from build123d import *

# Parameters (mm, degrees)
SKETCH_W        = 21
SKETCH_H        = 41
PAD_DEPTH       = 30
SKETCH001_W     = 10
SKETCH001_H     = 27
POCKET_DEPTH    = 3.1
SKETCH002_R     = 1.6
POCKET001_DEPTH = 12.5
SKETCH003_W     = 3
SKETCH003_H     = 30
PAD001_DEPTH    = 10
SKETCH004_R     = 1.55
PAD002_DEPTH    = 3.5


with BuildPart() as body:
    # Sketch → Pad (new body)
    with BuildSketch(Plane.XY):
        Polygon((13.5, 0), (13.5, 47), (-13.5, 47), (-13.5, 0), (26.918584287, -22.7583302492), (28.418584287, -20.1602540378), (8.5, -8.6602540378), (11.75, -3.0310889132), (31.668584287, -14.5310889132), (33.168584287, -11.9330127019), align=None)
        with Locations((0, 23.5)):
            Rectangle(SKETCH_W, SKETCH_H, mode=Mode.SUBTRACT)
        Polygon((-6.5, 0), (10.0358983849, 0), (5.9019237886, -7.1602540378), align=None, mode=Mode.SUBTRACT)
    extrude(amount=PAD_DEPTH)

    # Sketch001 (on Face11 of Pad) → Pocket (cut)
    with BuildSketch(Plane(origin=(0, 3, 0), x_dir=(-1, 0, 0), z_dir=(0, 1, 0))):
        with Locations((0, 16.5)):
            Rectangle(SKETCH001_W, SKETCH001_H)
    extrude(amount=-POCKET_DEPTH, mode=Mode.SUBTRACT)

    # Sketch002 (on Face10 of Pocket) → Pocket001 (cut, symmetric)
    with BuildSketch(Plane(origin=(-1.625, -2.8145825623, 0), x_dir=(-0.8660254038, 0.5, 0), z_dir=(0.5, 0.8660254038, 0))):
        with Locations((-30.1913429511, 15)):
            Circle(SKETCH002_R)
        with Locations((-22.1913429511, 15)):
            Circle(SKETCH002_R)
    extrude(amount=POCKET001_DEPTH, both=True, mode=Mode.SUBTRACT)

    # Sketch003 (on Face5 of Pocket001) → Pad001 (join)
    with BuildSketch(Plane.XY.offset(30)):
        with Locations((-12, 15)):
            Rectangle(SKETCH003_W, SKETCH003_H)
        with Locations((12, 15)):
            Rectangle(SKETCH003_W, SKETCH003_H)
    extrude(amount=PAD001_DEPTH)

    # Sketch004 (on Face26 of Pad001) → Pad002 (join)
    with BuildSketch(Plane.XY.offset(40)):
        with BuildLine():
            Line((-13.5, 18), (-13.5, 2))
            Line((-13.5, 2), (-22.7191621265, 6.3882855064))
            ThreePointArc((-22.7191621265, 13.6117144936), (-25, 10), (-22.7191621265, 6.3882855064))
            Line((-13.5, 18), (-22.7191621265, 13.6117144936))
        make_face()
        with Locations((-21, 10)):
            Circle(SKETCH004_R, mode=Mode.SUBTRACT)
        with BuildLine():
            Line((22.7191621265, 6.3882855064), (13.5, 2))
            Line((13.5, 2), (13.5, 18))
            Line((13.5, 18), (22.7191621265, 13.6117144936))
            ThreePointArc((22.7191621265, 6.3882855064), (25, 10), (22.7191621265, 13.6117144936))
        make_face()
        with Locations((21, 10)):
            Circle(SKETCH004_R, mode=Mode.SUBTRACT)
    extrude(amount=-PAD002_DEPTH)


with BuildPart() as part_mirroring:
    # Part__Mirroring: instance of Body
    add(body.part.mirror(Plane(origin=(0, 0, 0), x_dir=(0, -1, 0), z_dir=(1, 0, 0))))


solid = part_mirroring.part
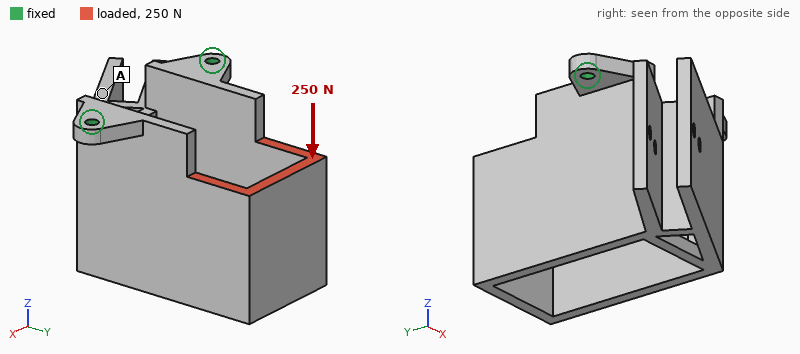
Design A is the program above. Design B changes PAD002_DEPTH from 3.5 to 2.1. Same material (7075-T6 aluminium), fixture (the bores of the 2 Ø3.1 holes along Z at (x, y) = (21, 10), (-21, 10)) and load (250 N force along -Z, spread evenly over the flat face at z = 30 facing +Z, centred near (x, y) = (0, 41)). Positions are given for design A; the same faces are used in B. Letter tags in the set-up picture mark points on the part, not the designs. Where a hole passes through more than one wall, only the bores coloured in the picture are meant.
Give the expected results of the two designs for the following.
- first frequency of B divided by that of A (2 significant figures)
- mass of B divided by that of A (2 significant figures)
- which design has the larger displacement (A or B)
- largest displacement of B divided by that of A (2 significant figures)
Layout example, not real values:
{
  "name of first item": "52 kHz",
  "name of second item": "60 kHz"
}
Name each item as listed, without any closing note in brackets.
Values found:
{
  "first frequency of B divided by that of A": "0.54",
  "mass of B divided by that of A": "0.99",
  "which design has the larger displacement": "B",
  "largest displacement of B divided by that of A": "3.3"
}
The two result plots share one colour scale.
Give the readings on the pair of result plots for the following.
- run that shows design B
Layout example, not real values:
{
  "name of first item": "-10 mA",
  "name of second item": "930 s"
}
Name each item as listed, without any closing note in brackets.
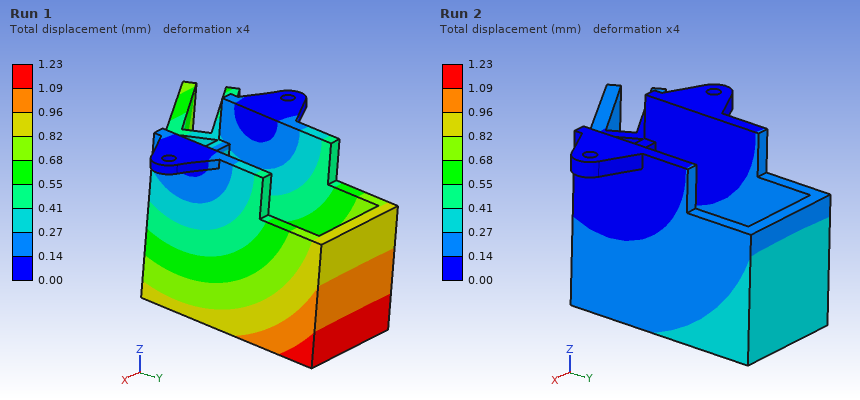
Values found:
{
  "run that shows design B": "Run 1"
}
